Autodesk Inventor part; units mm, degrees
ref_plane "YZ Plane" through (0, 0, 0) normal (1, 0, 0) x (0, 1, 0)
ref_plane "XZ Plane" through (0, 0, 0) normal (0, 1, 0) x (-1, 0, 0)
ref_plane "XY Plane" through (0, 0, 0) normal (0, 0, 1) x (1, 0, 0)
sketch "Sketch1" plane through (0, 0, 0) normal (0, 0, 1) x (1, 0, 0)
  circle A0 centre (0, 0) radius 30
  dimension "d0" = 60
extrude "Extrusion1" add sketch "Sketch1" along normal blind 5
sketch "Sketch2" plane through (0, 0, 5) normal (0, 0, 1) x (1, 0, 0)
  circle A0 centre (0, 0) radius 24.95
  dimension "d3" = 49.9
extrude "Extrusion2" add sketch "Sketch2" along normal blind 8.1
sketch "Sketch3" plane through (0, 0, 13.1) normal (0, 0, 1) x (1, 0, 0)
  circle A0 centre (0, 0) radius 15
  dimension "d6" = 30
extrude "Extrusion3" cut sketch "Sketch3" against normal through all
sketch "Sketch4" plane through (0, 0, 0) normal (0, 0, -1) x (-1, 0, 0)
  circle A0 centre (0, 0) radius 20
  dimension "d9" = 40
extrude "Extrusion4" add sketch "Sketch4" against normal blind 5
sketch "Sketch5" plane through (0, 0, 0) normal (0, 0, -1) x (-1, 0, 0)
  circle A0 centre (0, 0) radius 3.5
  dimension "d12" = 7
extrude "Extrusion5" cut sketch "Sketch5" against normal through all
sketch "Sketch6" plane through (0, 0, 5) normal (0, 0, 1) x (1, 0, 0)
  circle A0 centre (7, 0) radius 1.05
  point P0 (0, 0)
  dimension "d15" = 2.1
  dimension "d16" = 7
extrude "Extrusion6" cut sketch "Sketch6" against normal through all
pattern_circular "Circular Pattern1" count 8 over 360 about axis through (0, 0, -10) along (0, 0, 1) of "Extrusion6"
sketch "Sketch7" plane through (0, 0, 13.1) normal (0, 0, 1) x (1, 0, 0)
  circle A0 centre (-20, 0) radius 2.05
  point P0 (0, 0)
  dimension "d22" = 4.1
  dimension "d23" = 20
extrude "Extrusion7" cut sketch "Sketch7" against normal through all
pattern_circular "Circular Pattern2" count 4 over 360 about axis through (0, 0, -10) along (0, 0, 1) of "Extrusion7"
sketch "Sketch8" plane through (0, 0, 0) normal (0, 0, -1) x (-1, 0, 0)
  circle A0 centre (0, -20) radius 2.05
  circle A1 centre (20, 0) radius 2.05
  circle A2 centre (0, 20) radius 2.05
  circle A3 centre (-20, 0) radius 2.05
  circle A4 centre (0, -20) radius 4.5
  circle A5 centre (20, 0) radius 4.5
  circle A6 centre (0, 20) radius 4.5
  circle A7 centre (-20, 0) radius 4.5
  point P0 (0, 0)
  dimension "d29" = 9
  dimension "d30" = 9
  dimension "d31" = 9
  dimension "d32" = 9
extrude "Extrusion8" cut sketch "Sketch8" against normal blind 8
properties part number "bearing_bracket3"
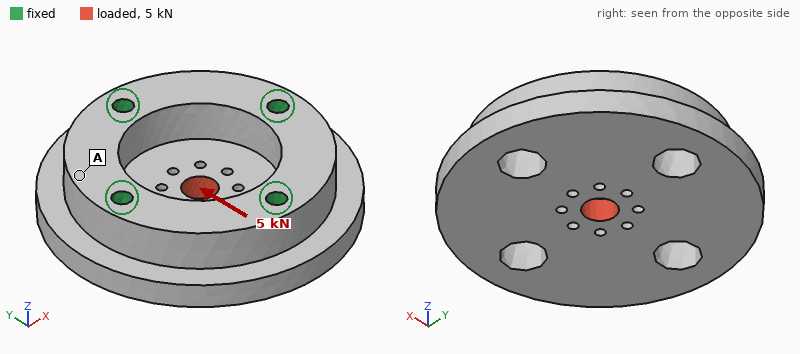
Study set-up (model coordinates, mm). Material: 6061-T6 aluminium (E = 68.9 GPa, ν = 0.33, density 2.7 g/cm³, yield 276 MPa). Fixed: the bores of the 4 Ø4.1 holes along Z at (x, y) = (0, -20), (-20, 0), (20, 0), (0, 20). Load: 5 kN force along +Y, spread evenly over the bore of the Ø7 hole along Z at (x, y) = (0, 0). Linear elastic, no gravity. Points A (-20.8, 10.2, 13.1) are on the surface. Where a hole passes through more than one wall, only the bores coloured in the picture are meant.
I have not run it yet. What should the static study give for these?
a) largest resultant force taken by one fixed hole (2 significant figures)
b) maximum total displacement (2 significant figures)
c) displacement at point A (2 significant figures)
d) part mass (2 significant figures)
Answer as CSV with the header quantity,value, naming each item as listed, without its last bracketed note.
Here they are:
quantity,value
largest resultant force taken by one fixed hole,1.5 kN
maximum total displacement,16 µm
displacement at point A,3.2 µm
part mass,58 g
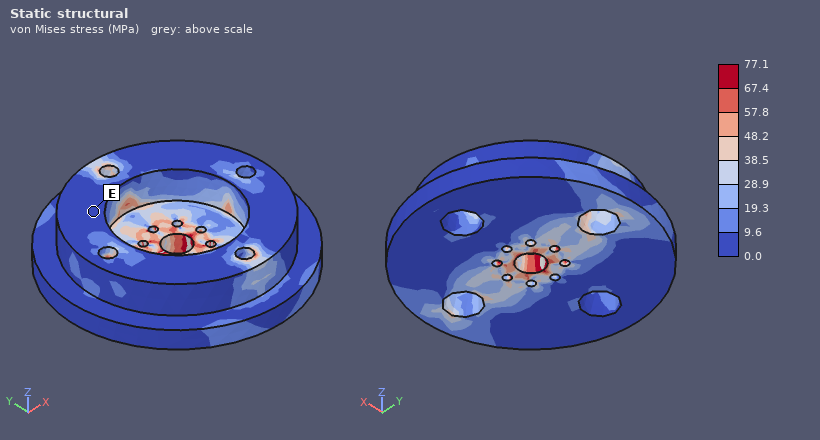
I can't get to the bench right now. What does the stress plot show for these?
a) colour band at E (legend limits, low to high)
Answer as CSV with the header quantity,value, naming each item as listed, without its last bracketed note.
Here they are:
quantity,value
colour band at E,0.0 to 9.6 MPa
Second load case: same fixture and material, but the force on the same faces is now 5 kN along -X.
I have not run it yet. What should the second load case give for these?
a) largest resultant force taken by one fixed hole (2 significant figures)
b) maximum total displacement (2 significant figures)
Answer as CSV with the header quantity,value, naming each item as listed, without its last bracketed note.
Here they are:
quantity,value
largest resultant force taken by one fixed hole,1.5 kN
maximum total displacement,16 µm
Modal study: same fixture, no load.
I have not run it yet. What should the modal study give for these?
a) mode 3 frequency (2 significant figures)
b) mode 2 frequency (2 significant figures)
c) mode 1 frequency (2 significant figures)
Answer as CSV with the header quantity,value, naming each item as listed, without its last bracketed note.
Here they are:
quantity,value
mode 3 frequency,20 kHz
mode 2 frequency,18 kHz
mode 1 frequency,18 kHz
